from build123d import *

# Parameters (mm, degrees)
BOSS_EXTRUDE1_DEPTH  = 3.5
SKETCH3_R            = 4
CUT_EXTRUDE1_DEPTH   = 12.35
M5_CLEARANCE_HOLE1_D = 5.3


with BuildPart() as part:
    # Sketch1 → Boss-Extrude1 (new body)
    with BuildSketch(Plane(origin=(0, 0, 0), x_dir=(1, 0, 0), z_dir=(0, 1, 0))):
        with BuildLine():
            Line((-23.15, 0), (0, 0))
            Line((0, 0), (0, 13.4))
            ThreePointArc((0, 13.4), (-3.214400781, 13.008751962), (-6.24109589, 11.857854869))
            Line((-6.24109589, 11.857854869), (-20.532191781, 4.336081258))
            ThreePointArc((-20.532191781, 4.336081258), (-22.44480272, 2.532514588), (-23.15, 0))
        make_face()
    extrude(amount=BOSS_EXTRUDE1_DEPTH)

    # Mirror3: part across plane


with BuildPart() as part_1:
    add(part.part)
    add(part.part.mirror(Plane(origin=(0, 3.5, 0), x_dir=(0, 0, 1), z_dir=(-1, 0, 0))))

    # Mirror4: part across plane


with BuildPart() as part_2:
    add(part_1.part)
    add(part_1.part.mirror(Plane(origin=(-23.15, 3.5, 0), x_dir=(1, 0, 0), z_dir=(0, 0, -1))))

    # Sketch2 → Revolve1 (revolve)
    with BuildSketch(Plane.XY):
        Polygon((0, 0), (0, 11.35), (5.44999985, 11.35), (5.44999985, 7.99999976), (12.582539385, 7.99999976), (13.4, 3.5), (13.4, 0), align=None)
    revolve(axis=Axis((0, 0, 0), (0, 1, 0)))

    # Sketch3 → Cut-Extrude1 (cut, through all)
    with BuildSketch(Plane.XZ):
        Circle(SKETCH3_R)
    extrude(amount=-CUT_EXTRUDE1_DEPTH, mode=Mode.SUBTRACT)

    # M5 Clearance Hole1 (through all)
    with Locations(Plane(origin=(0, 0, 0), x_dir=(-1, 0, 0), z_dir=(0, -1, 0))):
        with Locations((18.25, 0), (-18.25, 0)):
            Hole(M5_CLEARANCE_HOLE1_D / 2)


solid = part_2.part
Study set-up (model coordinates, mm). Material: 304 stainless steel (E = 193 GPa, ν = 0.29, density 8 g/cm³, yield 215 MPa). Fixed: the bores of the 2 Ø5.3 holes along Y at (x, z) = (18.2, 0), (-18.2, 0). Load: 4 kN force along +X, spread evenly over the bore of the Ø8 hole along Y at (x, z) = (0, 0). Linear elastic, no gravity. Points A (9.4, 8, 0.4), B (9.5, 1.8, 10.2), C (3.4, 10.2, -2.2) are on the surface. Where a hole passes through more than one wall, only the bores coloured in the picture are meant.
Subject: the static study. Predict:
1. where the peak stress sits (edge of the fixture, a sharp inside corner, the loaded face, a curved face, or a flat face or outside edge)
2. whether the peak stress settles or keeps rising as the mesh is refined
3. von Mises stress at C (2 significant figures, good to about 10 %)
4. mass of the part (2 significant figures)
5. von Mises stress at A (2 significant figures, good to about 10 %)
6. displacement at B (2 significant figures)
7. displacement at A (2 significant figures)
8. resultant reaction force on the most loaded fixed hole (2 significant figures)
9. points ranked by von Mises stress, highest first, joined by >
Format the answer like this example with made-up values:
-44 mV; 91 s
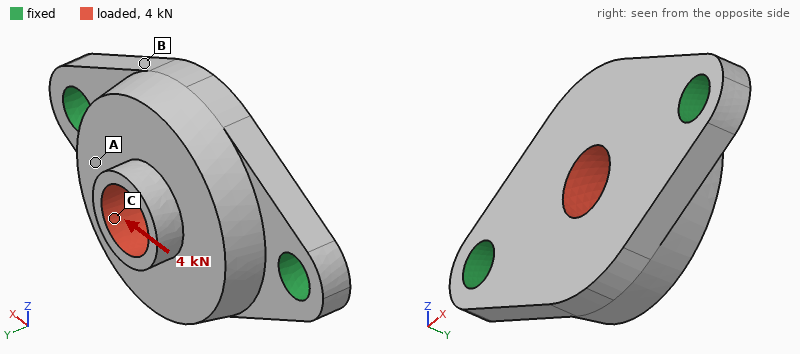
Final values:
edge of the fixture; keeps rising; 44 MPa; 39 g; 16 MPa; 2.0 µm; 2.6 µm; 2.1 kN; C > A > B
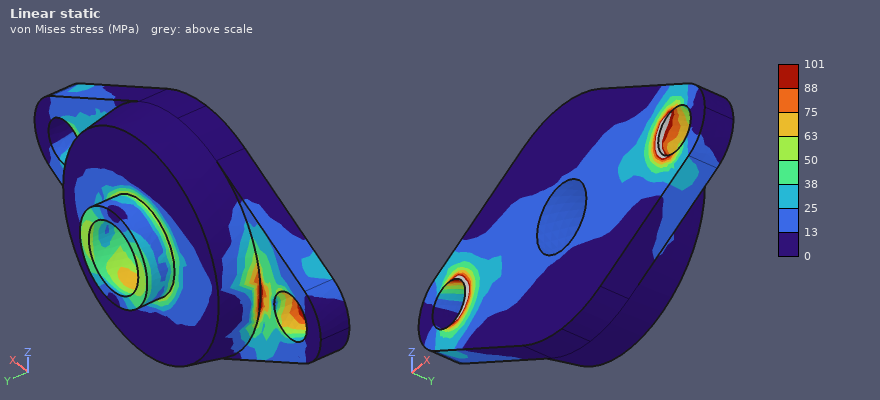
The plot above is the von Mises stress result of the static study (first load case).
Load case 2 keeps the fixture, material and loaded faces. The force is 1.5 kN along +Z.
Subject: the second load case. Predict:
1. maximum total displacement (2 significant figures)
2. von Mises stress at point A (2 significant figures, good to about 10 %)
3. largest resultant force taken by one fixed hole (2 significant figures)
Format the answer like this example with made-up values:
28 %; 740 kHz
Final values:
13 µm; 19 MPa; 750 N
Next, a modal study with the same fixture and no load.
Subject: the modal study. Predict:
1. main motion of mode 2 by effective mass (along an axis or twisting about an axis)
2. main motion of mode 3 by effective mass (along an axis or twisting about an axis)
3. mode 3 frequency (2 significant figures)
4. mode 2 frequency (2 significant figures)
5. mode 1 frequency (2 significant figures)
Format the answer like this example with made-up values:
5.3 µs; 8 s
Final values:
along Y; along Z; 26 kHz; 15 kHz; 9400 Hz
